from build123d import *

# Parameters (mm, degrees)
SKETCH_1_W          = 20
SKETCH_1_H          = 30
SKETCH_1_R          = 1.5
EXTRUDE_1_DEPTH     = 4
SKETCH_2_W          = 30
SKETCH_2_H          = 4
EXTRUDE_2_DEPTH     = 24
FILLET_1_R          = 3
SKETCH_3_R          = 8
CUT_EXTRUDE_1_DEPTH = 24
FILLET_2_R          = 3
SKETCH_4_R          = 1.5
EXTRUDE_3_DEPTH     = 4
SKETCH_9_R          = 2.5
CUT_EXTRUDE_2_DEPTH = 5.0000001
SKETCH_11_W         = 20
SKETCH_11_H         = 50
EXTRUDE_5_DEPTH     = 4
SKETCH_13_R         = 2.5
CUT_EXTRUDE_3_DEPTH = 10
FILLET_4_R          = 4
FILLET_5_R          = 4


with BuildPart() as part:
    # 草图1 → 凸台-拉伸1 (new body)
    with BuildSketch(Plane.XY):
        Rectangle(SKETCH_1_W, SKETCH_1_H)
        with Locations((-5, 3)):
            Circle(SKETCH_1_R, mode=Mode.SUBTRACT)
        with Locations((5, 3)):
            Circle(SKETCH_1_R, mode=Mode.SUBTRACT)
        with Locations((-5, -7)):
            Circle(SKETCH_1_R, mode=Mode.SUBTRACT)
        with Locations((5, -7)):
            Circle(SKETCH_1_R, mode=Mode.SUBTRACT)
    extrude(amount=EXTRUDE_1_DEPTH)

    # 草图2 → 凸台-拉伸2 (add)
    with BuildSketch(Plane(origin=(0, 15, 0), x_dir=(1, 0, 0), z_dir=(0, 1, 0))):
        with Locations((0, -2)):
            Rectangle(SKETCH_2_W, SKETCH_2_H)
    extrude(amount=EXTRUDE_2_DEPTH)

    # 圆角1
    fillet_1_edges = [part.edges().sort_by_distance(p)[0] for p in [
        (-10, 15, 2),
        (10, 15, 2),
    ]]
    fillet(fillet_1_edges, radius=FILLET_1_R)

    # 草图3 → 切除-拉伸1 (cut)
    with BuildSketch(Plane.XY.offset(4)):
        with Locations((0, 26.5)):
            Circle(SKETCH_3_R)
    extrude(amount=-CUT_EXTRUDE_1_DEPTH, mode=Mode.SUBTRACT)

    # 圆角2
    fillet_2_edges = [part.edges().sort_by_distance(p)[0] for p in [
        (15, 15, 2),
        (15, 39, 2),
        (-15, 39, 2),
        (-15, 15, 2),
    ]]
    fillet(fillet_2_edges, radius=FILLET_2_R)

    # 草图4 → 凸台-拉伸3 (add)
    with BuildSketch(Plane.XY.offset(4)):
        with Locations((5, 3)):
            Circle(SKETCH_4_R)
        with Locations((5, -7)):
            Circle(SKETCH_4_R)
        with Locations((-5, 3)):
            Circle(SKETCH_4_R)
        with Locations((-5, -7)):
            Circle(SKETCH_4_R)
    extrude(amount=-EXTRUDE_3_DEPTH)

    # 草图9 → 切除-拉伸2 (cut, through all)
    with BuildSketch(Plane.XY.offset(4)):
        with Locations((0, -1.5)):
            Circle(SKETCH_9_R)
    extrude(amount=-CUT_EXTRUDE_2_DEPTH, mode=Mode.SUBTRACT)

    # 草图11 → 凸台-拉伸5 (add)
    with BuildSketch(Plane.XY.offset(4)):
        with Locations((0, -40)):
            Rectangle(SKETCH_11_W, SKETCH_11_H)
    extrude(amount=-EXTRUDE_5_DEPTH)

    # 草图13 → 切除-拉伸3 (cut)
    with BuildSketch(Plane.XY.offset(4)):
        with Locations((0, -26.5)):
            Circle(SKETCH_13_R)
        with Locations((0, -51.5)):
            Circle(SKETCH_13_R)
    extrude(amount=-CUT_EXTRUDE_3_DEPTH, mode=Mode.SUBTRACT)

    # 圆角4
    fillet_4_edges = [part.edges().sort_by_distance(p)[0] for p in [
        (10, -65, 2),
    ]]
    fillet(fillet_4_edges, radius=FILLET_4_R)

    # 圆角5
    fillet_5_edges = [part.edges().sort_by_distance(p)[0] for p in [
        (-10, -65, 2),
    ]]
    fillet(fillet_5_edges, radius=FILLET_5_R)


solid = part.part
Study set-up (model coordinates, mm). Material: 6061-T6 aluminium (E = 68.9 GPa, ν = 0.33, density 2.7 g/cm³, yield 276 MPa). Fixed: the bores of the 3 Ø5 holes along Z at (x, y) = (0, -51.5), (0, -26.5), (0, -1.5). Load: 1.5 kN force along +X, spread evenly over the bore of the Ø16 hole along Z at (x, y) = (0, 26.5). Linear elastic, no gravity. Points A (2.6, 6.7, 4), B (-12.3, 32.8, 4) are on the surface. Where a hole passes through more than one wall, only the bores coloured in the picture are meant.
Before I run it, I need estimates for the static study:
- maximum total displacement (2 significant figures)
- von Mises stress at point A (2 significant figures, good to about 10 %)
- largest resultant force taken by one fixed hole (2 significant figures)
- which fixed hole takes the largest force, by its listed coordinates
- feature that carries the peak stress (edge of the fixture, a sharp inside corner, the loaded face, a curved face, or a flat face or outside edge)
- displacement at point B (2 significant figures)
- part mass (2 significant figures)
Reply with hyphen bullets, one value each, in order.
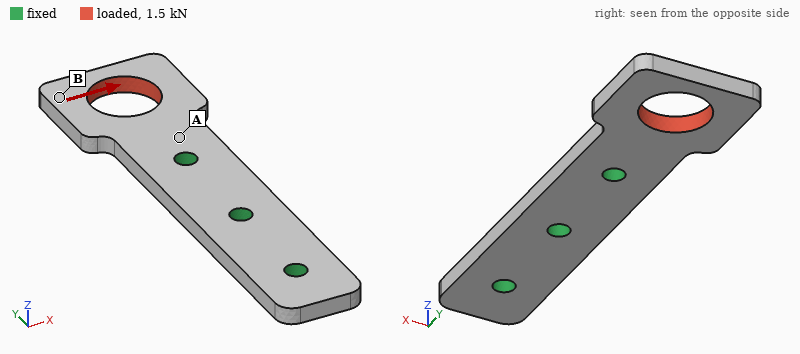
- 0.25 mm
- 56 MPa
- 2.5 kN
- (0, -1.5)
- edge of the fixture
- 0.21 mm
- 22 g
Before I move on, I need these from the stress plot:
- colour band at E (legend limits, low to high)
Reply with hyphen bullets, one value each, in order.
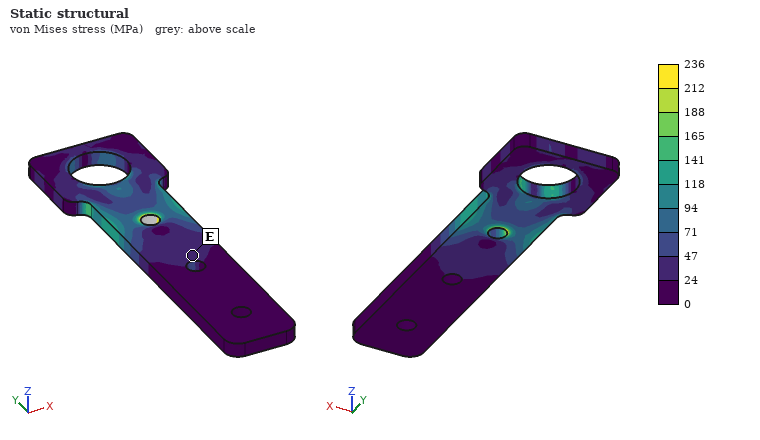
- 24 to 47 MPa
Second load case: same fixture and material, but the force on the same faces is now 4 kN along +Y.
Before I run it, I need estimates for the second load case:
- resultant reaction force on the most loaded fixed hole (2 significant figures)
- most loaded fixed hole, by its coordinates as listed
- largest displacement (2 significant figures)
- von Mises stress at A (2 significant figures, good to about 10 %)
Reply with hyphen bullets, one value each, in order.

- 3.5 kN
- (0, -1.5)
- 58 µm
- 53 MPa
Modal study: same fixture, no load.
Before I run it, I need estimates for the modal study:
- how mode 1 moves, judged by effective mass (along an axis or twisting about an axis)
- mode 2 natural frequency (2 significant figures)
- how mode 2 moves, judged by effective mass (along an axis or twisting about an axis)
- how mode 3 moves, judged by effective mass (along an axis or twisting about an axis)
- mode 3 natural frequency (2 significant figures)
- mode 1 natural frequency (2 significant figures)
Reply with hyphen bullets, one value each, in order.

- along Z
- 4200 Hz
- twisting about Y
- along X
- 5700 Hz
- 1900 Hz
